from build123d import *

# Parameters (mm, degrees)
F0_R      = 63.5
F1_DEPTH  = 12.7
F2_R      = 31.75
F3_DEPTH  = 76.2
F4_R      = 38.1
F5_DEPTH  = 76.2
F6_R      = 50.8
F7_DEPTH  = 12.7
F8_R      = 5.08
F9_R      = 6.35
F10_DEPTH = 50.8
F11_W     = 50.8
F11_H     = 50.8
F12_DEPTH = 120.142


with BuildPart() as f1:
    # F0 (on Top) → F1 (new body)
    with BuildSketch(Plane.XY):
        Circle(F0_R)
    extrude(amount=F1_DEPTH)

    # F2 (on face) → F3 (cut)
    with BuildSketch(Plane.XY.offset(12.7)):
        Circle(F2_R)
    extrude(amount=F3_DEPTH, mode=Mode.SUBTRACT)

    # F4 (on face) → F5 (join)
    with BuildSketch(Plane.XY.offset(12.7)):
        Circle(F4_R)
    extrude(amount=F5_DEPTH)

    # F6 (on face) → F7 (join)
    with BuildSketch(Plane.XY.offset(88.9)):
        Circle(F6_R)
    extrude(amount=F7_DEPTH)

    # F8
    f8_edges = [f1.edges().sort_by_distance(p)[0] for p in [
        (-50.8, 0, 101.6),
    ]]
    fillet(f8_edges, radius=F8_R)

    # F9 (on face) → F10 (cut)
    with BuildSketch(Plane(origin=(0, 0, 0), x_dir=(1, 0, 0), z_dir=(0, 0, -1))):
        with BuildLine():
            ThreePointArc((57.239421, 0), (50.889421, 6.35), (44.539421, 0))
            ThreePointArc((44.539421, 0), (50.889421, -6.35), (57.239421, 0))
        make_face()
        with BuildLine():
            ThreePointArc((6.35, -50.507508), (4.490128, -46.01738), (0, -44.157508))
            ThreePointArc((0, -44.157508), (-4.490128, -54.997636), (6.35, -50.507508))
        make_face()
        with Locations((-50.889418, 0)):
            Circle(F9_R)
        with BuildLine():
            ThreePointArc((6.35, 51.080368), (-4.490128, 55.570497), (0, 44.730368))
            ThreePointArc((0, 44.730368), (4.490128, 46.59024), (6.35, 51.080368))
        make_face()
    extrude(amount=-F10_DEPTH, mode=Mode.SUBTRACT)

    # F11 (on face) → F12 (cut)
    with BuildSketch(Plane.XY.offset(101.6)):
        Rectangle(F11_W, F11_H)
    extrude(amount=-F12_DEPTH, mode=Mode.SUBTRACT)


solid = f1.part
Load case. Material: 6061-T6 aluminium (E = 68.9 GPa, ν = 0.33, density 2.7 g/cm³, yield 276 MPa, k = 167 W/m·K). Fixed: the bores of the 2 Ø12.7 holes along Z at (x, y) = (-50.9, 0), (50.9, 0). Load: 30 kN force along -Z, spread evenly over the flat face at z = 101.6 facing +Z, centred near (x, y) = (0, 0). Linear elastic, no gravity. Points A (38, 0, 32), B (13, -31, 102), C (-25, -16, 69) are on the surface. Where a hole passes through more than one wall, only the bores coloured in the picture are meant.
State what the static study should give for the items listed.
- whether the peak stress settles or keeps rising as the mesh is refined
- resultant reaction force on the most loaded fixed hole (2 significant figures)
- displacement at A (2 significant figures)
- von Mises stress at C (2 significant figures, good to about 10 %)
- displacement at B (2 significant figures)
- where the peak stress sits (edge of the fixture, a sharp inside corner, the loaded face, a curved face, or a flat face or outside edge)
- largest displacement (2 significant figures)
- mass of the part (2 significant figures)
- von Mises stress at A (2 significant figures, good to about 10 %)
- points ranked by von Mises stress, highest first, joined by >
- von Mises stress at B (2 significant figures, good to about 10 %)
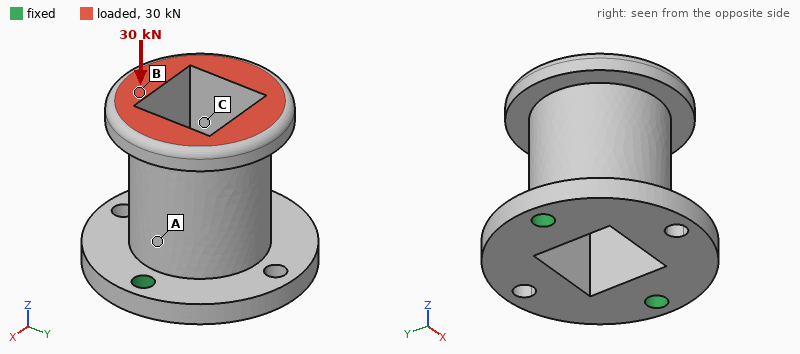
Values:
keeps rising
15 kN
53 µm
24 MPa
73 µm
edge of the fixture
83 µm
920 g
44 MPa
A > C > B
12 MPa
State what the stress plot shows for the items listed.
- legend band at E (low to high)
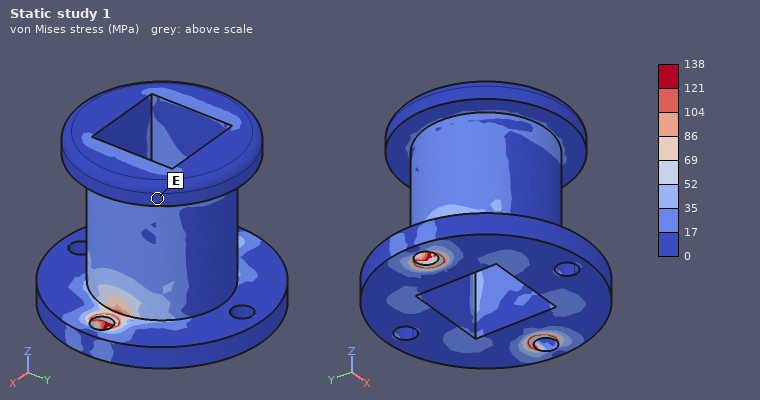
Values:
0 to 17 MPa
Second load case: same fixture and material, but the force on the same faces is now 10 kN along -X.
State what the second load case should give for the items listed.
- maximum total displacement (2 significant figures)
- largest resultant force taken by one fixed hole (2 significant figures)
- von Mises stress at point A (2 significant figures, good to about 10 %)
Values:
0.17 mm
13 kN
37 MPa
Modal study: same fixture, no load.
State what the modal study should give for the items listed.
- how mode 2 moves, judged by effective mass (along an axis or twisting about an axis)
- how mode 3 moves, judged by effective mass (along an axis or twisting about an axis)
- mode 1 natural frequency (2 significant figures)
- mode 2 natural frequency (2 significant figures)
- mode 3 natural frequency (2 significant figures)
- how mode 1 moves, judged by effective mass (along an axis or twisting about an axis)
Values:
along X
along Z
930 Hz
2400 Hz
3700 Hz
along Y
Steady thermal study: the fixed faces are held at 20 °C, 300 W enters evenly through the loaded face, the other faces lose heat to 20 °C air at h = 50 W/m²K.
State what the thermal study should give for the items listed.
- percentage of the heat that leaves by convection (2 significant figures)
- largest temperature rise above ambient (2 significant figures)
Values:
43 %
76 K
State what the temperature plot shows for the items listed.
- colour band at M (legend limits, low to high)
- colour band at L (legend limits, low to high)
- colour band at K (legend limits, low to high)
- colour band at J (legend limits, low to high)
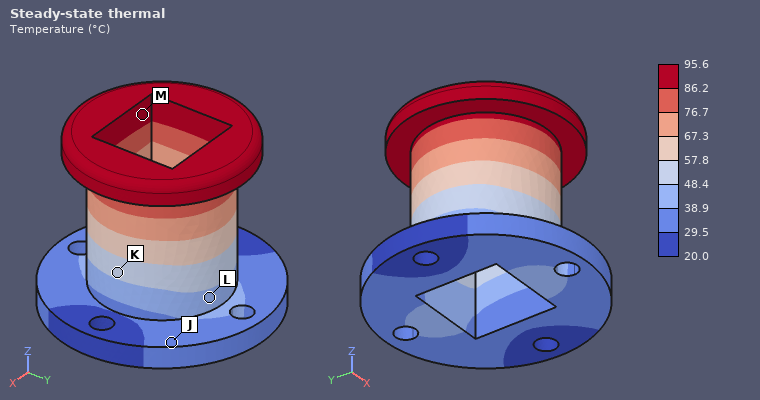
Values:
86.2 to 95.6 °C
38.9 to 48.4 °C
48.4 to 57.8 °C
29.5 to 38.9 °C
